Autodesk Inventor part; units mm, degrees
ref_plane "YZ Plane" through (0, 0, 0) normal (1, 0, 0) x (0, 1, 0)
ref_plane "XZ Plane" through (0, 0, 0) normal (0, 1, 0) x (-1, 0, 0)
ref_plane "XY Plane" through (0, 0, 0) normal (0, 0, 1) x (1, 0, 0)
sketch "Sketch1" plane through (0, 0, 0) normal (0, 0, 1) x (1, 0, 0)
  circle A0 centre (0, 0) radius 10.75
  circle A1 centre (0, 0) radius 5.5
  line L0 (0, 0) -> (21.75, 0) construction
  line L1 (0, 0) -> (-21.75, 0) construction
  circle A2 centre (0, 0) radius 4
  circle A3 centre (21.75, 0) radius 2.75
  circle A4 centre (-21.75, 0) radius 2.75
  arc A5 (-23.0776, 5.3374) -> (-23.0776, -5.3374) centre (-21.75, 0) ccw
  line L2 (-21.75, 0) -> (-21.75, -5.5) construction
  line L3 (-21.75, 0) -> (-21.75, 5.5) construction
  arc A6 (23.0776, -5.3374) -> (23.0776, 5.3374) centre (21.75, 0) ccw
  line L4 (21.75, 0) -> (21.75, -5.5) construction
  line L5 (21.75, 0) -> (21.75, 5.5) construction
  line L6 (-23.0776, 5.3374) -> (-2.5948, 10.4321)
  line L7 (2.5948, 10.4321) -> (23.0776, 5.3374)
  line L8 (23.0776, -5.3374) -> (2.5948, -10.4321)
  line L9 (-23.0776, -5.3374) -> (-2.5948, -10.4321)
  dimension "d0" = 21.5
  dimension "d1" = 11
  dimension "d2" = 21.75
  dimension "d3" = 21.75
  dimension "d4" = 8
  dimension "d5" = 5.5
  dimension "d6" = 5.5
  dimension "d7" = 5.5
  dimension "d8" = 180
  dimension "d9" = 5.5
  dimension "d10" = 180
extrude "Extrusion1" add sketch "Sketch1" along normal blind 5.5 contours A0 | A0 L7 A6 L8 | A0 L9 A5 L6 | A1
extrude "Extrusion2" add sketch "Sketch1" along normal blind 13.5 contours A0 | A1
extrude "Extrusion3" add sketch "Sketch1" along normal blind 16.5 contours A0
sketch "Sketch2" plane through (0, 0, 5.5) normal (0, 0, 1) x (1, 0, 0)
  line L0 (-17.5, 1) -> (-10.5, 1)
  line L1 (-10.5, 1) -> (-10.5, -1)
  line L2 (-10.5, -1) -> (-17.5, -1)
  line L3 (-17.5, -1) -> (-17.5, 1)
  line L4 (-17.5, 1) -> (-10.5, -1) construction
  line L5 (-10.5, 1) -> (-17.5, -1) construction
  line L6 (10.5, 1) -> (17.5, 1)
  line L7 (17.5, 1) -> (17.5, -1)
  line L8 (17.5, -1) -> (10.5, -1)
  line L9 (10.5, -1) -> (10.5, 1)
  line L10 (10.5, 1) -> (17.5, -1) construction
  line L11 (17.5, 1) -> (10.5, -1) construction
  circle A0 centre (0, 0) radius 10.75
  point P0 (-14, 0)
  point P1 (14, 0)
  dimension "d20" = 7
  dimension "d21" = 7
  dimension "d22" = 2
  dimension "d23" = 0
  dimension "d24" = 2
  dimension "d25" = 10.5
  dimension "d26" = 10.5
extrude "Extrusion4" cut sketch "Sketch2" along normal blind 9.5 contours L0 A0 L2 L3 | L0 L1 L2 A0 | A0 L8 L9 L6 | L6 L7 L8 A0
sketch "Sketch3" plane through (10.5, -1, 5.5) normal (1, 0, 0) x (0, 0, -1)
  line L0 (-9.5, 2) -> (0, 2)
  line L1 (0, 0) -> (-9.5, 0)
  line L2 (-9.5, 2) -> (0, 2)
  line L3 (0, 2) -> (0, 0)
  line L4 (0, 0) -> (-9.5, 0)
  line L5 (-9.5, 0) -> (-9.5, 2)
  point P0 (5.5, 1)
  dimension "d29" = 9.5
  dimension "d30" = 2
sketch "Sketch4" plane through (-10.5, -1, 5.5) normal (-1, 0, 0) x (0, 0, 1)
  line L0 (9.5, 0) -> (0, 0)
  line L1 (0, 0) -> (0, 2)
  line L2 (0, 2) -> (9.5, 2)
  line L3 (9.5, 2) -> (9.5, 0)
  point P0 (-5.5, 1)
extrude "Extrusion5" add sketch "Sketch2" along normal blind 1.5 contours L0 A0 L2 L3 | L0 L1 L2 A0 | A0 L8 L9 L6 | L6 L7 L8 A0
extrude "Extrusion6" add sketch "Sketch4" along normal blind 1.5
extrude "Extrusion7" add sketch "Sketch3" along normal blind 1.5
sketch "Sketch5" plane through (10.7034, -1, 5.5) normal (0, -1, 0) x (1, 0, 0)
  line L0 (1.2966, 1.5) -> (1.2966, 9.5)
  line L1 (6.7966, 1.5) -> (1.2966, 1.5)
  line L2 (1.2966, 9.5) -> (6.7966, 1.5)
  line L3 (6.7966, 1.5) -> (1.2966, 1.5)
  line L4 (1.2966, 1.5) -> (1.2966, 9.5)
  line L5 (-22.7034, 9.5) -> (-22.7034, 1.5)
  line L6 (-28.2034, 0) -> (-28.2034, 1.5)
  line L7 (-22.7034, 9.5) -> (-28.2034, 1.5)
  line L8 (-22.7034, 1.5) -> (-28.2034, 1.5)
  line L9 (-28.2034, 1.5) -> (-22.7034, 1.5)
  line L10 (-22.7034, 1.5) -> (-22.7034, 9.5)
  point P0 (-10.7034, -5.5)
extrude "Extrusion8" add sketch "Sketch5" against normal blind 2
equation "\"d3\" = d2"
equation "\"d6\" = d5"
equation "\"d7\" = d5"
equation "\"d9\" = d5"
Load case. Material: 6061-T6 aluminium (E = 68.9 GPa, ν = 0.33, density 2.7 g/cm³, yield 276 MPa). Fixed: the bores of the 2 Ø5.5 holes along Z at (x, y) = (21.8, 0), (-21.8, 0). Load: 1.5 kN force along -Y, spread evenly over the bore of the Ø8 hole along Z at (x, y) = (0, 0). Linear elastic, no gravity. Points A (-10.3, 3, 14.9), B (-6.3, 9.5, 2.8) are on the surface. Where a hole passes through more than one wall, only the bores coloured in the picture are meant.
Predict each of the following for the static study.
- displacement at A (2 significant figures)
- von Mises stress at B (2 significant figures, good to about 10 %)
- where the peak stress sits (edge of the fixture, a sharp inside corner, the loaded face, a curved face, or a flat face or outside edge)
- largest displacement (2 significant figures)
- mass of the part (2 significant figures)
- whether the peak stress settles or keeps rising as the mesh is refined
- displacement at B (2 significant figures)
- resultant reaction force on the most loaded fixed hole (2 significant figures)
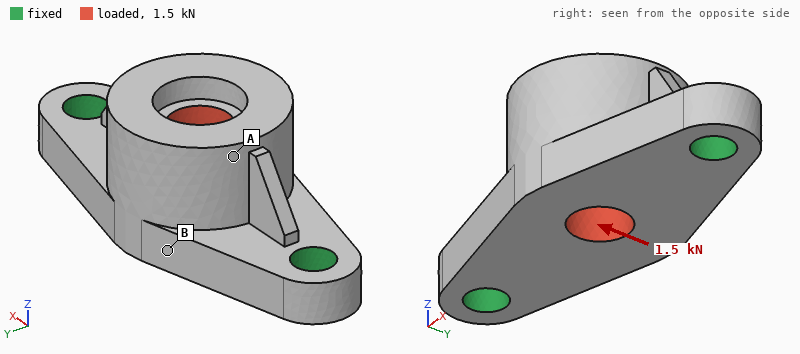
31 µm
22 MPa
edge of the fixture
39 µm
20 g
keeps rising
18 µm
750 N
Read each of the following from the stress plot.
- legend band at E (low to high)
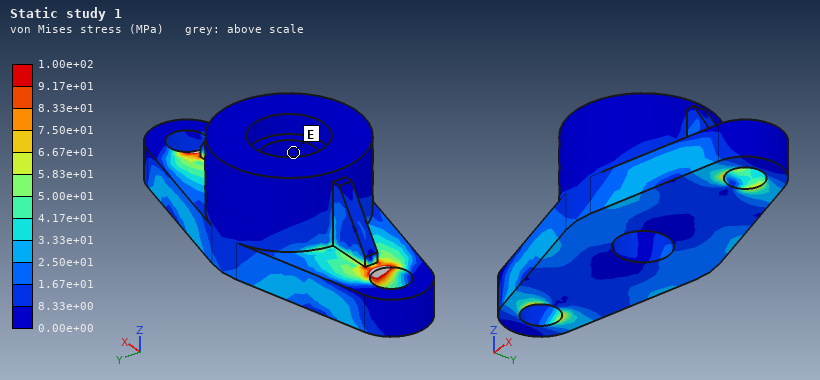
0.00e+00 to 8.33e+00 MPa
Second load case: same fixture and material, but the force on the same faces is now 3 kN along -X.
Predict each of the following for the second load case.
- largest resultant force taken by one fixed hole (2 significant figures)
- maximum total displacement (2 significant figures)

1.5 kN
6.8 µm
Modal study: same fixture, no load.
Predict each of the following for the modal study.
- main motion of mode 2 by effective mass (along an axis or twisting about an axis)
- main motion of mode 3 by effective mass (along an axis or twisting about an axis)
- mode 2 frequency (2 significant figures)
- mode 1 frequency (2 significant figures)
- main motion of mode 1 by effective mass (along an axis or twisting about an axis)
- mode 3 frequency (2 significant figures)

along Z
along Y
14 kHz
8000 Hz
along Y
21 kHz
